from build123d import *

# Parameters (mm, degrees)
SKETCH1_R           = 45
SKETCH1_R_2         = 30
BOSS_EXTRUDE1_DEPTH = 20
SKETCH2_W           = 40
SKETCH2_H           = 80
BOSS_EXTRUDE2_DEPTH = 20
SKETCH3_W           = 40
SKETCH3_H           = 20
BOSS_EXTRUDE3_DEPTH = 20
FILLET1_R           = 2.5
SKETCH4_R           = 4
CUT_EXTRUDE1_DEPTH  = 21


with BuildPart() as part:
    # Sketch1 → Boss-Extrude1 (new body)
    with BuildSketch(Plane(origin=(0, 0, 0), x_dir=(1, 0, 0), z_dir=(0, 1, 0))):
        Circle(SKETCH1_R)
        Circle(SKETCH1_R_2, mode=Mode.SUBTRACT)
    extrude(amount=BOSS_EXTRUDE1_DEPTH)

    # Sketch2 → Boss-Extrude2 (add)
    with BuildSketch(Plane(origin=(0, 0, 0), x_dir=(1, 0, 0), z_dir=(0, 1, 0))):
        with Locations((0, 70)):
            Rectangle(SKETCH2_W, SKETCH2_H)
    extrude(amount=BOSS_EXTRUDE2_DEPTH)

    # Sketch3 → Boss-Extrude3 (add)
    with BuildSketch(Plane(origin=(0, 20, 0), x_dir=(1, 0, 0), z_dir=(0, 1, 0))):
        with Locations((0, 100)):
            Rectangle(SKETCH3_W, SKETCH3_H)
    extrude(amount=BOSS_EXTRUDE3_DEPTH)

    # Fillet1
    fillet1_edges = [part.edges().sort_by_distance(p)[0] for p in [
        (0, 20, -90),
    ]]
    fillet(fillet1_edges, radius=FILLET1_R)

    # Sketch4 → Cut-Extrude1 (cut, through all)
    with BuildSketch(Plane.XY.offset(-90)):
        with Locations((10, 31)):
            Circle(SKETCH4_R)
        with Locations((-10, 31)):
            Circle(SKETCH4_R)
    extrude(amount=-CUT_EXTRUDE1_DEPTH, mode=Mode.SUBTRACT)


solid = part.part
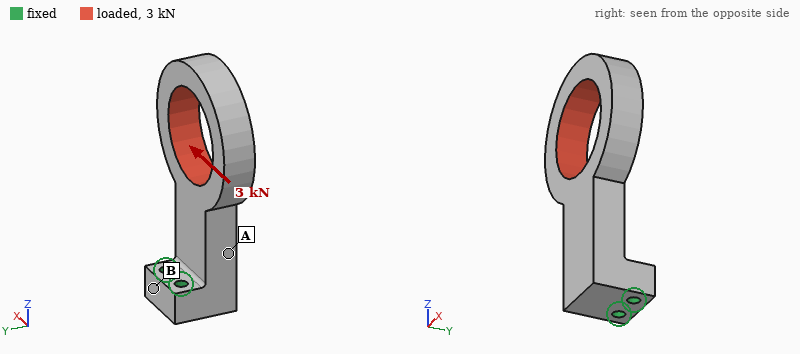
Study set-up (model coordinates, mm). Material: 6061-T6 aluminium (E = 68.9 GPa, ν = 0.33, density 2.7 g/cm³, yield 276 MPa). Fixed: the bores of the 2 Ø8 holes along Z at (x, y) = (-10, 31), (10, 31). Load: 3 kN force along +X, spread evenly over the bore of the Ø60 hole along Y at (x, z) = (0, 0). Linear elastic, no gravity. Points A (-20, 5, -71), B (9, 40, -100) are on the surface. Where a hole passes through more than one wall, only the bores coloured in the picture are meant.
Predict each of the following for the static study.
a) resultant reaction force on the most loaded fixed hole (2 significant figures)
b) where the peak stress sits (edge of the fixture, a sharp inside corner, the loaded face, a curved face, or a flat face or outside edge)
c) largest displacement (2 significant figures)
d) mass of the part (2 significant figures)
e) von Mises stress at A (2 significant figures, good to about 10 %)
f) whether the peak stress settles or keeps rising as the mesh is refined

9.0 kN
edge of the fixture
0.56 mm
370 g
38 MPa
keeps rising
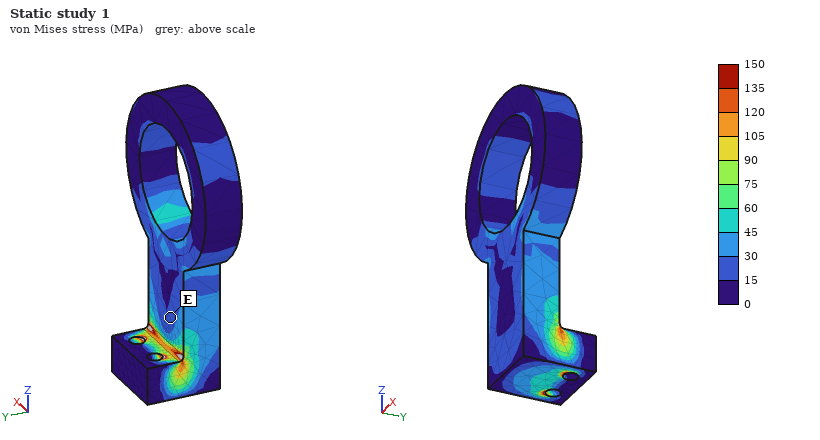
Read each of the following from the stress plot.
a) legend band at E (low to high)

15 to 30 MPa
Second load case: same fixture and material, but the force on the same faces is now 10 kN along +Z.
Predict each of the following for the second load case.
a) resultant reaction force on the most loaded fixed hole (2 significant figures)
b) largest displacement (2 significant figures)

5.0 kN
0.22 mm
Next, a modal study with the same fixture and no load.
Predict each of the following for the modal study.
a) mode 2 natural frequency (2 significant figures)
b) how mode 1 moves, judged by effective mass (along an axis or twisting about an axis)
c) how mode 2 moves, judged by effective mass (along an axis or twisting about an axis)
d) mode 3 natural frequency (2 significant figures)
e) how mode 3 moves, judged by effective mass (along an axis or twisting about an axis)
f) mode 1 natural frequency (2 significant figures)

940 Hz
along Y
along X
1900 Hz
twisting about Z
640 Hz
